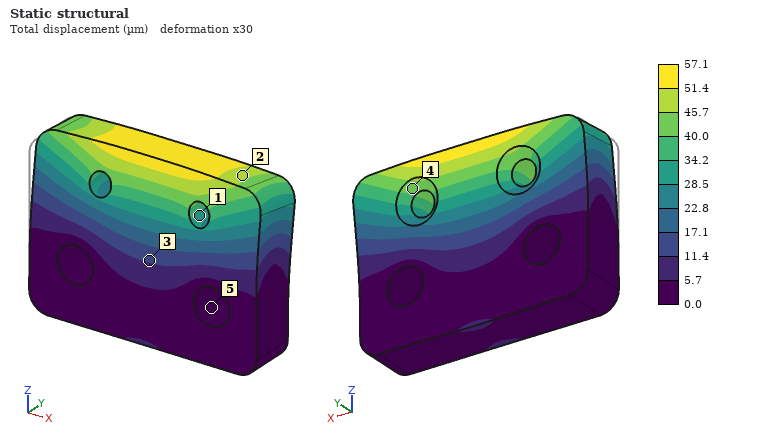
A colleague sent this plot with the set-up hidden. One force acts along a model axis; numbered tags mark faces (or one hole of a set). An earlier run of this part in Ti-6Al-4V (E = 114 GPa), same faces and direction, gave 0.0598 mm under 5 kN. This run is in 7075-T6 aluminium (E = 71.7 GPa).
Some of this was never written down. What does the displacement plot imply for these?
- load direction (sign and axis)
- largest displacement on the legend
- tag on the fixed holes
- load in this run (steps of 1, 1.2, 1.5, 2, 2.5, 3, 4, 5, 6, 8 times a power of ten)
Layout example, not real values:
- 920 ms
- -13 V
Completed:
- +Y
- 57.1 µm
- 5
- 3 kN
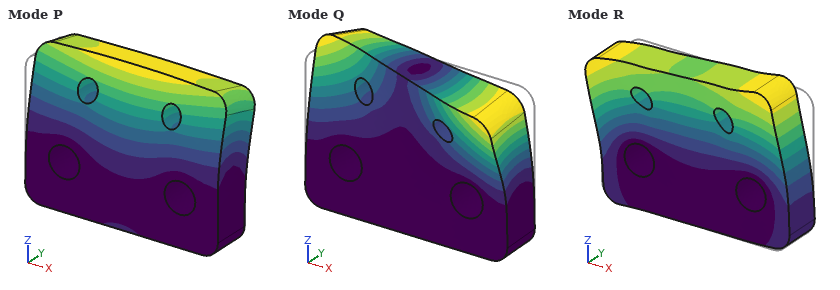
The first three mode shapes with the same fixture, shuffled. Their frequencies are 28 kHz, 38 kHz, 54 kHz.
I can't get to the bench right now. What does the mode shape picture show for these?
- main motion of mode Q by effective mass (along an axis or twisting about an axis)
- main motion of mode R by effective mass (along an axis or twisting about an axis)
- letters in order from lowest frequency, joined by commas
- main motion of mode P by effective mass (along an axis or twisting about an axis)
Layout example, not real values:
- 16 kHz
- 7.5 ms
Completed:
- twisting about Z
- along X
- P, Q, R
- along Y
